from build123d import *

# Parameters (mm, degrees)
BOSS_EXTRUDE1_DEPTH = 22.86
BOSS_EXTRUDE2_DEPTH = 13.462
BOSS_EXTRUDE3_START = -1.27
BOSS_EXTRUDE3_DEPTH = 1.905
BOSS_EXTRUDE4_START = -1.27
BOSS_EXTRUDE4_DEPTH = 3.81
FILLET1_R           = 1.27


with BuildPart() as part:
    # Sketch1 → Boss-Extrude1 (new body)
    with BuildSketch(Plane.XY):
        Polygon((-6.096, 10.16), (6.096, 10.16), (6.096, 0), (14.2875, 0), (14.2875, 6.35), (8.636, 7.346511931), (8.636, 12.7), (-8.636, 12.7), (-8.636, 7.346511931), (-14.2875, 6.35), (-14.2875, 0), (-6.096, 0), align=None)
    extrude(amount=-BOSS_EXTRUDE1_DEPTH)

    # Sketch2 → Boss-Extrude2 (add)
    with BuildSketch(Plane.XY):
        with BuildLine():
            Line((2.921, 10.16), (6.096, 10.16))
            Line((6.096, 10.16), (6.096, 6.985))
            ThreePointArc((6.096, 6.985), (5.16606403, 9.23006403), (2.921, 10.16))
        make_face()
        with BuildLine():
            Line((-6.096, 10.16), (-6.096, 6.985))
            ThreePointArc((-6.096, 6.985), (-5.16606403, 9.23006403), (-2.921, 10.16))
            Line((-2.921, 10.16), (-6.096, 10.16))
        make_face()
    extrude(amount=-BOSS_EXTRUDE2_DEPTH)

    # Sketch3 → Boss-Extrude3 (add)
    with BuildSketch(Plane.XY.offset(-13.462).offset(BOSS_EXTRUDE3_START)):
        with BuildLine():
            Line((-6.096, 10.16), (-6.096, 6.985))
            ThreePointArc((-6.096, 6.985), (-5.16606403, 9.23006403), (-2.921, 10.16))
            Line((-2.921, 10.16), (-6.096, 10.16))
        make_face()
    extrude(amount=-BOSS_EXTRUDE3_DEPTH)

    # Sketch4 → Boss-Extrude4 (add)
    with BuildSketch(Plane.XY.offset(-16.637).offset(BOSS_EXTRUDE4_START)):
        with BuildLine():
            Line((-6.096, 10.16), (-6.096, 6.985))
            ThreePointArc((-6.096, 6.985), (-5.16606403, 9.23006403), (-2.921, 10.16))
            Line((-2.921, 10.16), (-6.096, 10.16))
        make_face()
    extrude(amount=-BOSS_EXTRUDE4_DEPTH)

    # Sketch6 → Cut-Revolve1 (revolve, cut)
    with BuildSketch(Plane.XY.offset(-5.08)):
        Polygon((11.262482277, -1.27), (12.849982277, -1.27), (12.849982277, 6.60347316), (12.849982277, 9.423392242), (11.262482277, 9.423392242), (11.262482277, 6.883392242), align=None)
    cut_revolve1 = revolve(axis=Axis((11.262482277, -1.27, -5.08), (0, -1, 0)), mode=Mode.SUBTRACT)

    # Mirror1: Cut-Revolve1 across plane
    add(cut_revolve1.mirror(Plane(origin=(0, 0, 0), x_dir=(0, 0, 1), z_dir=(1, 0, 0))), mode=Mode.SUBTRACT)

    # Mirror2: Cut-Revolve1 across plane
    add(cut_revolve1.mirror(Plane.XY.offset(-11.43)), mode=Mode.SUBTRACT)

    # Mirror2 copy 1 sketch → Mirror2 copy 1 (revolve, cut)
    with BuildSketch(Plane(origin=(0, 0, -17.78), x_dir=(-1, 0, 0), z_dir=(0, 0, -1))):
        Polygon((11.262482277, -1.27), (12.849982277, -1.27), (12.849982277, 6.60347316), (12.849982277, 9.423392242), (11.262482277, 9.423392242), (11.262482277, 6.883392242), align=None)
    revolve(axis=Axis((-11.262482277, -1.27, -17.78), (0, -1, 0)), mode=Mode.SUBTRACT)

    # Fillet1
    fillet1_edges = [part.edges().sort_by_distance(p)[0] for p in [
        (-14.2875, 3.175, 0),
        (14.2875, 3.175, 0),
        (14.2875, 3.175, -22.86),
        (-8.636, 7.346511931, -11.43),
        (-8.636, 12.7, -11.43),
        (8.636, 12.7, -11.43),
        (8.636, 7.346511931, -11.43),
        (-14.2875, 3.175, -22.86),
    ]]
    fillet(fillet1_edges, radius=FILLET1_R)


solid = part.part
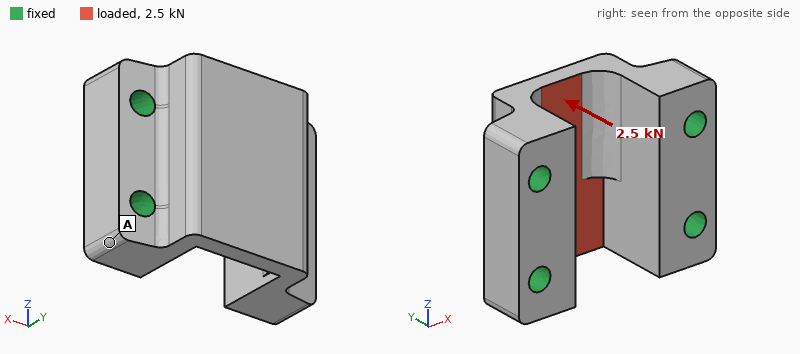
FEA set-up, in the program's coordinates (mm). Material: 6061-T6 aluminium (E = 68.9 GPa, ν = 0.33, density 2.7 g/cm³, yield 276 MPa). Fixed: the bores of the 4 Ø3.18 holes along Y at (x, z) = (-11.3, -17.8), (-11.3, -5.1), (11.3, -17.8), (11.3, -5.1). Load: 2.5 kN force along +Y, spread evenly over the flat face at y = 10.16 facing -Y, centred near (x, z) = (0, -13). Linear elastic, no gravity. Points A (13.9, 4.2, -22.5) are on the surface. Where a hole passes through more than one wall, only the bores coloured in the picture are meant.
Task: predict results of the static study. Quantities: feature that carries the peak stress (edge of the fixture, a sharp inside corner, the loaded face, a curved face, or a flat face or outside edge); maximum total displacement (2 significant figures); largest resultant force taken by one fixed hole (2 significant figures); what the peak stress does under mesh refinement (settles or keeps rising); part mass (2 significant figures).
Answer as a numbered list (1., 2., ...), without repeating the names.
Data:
1. a sharp inside corner
2. 25 µm
3. 950 N
4. keeps rising
5. 10 g
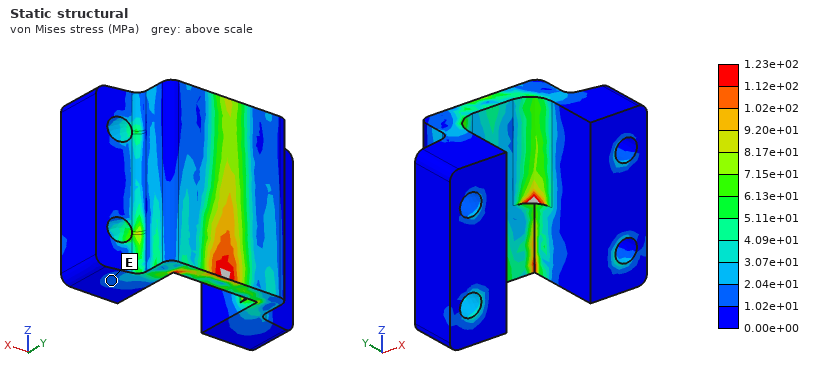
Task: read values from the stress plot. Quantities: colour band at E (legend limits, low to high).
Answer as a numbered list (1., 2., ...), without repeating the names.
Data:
1. 1.02e+01 to 2.04e+01 MPa
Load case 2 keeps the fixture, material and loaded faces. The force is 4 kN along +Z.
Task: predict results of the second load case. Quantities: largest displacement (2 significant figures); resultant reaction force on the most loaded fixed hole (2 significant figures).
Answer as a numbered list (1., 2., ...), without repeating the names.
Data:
1. 23 µm
2. 1.3 kN
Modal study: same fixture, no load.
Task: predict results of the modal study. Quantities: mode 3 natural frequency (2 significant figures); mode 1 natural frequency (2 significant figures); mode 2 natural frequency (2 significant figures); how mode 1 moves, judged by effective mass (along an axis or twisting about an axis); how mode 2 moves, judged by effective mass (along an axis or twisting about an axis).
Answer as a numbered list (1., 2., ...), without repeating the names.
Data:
1. 50 kHz
2. 40 kHz
3. 46 kHz
4. along X
5. along Z
